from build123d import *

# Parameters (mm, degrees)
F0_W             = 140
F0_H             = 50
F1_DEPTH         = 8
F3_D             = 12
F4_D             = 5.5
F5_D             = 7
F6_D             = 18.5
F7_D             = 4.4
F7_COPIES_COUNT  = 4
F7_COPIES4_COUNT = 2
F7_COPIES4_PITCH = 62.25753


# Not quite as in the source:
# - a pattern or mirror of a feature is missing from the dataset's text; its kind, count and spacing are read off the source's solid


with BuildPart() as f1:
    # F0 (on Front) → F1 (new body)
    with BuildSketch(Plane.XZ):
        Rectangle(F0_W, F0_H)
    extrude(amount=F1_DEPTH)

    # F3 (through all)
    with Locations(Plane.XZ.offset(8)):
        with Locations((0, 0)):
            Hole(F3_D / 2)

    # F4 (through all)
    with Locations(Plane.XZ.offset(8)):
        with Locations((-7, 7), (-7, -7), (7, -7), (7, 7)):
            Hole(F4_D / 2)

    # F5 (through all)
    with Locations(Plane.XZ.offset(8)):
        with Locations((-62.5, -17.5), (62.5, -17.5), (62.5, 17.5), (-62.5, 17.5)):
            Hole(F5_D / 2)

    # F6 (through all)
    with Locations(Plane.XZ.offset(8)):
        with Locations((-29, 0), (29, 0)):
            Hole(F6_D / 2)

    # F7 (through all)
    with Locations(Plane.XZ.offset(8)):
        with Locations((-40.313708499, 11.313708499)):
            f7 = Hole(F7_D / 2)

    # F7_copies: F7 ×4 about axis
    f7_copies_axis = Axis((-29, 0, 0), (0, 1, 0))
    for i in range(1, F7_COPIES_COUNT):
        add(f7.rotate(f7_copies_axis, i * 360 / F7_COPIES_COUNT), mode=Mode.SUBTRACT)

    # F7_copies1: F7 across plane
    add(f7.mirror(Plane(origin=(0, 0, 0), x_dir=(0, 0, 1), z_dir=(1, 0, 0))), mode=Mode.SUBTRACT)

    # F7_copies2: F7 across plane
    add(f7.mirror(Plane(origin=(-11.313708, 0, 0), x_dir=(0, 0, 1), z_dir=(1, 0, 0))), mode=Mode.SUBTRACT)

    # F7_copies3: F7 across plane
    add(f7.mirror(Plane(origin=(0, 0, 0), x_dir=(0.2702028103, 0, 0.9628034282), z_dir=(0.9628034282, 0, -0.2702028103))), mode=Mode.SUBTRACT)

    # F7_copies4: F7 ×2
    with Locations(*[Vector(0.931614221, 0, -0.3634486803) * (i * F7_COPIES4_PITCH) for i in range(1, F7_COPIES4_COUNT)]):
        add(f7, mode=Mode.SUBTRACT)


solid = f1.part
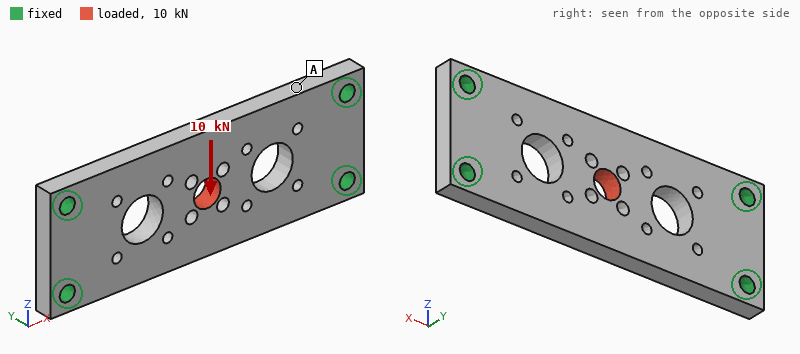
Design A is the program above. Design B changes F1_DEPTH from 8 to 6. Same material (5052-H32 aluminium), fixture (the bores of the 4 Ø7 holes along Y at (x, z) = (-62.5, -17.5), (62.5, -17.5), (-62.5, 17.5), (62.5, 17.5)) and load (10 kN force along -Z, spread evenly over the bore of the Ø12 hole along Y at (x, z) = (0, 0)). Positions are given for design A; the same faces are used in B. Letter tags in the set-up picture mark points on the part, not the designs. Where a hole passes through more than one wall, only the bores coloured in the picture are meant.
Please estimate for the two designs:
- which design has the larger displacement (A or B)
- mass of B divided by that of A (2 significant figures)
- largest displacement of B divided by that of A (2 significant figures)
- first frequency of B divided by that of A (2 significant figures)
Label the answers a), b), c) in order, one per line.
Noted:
a) B
b) 0.75
c) 1.3
d) 0.77
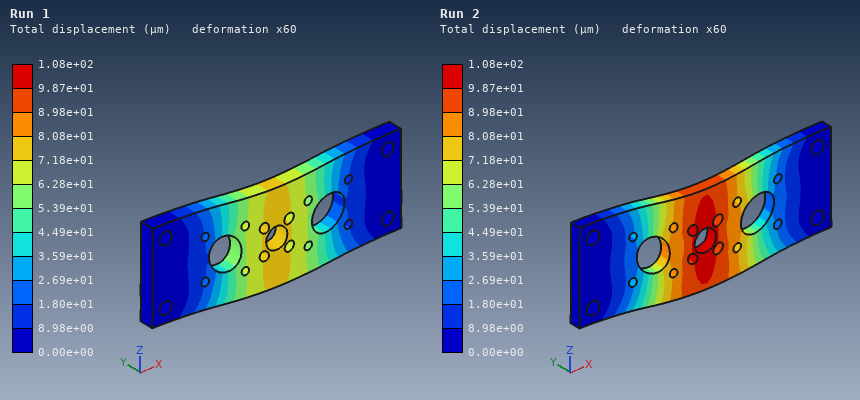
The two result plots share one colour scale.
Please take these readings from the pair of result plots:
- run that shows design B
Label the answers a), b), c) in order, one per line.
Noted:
a) Run 2
